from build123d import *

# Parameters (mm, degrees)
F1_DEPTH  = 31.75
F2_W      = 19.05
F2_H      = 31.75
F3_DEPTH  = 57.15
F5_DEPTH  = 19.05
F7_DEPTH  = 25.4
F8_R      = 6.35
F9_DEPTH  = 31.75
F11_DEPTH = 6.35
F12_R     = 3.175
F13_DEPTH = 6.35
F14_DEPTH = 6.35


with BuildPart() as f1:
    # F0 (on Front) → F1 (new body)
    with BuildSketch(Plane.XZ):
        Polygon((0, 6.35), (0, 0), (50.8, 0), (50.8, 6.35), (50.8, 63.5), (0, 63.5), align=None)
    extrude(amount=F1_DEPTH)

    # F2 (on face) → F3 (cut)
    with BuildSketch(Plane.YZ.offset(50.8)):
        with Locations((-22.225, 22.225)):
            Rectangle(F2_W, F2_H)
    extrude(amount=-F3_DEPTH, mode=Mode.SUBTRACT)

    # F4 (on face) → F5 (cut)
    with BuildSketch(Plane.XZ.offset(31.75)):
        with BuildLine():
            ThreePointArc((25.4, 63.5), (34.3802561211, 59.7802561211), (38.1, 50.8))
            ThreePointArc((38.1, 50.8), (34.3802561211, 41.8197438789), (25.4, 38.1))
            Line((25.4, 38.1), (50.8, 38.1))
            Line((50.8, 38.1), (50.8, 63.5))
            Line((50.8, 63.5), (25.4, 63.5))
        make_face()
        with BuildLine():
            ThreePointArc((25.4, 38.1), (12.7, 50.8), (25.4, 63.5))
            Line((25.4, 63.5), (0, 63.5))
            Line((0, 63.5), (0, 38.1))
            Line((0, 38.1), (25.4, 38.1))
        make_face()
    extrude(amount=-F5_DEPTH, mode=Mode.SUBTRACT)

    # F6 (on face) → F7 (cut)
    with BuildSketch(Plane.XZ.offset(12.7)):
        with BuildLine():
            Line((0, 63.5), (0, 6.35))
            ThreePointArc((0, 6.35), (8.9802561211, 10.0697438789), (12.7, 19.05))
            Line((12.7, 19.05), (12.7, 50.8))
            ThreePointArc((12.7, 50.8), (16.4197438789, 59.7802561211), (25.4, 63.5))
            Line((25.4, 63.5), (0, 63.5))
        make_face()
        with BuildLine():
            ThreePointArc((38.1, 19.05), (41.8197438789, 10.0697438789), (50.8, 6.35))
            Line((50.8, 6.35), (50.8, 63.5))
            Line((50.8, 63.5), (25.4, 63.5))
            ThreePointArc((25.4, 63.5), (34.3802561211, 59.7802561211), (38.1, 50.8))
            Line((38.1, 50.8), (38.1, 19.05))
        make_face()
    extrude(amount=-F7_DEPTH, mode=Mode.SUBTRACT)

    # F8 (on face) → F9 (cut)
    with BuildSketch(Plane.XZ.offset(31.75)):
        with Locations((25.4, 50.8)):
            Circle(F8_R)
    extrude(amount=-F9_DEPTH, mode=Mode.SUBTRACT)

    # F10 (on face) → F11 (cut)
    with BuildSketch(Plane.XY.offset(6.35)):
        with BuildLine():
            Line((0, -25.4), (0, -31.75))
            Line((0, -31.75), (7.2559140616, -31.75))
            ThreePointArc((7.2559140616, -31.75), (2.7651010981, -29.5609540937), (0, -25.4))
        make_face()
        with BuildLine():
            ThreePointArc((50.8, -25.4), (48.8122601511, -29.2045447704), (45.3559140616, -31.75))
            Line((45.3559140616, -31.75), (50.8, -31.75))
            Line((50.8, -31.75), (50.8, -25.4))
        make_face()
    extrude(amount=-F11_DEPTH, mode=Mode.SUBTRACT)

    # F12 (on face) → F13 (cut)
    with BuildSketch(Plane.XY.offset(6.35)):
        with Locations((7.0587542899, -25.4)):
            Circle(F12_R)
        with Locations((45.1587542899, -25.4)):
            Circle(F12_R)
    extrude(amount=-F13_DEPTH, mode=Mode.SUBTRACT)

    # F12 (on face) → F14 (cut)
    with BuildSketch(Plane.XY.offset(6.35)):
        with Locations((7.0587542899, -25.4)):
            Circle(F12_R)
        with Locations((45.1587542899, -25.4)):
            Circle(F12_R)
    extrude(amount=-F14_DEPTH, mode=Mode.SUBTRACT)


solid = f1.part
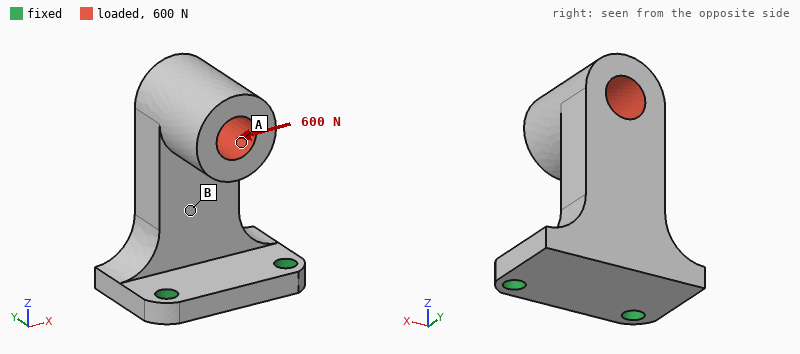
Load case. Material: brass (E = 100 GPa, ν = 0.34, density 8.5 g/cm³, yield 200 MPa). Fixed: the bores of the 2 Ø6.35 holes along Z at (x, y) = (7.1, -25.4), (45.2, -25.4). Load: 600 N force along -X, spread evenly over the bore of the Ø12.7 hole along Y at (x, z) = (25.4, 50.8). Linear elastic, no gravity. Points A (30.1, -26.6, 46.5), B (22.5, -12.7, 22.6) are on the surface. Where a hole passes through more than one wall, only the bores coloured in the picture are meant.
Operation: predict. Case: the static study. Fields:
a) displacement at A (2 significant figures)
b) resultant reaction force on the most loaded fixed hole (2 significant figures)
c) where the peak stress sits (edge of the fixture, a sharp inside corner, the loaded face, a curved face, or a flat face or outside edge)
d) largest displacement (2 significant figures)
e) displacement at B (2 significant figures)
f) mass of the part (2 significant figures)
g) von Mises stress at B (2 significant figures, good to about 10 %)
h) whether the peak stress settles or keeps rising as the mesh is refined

53 µm
830 N
edge of the fixture
73 µm
18 µm
290 g
16 MPa
keeps rising
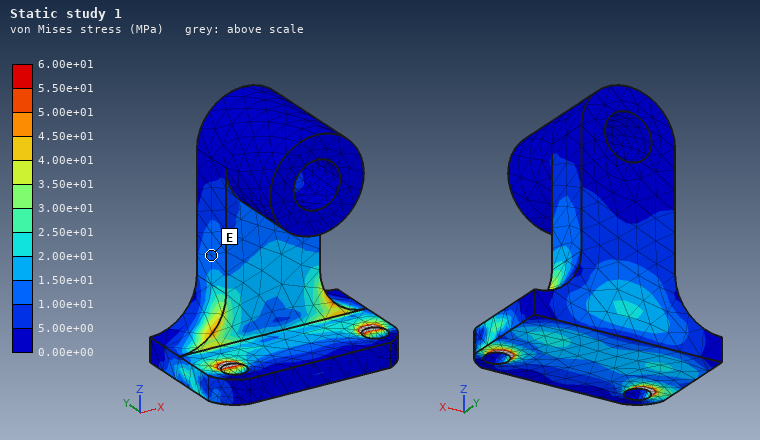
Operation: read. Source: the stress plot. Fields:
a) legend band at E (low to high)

1.00e+01 to 1.50e+01 MPa
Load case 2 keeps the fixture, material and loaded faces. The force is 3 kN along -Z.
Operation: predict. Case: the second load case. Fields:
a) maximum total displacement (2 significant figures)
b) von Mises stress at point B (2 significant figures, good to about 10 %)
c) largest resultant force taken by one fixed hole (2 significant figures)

91 µm
47 MPa
1.6 kN
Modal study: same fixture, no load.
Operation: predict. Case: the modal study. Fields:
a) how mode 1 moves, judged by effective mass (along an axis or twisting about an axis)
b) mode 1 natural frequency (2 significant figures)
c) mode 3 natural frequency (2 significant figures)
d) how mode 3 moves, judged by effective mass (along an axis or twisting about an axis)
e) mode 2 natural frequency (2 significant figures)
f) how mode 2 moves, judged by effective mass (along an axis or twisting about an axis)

along Y
680 Hz
2900 Hz
along Z
1500 Hz
along X
